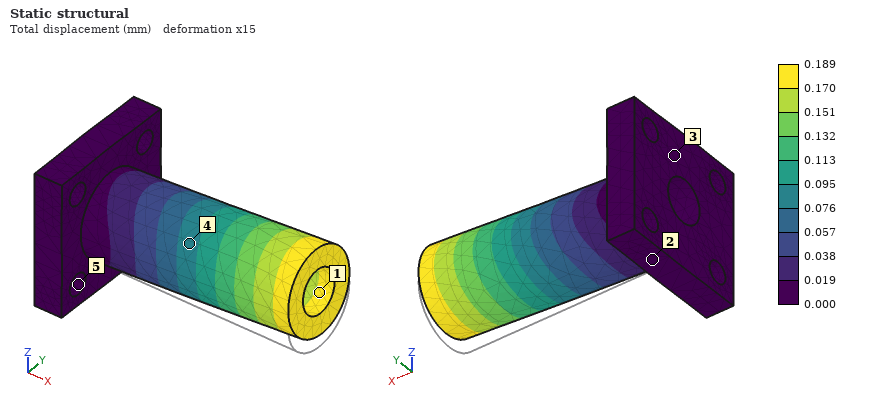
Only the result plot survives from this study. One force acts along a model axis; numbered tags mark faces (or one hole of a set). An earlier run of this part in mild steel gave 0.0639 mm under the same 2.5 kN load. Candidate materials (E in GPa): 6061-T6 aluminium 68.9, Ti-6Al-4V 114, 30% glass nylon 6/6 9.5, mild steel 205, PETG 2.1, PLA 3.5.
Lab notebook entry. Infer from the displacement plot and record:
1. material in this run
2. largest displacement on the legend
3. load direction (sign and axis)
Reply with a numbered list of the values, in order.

1. 6061-T6 aluminium
2. 0.189 mm
3. +Z
